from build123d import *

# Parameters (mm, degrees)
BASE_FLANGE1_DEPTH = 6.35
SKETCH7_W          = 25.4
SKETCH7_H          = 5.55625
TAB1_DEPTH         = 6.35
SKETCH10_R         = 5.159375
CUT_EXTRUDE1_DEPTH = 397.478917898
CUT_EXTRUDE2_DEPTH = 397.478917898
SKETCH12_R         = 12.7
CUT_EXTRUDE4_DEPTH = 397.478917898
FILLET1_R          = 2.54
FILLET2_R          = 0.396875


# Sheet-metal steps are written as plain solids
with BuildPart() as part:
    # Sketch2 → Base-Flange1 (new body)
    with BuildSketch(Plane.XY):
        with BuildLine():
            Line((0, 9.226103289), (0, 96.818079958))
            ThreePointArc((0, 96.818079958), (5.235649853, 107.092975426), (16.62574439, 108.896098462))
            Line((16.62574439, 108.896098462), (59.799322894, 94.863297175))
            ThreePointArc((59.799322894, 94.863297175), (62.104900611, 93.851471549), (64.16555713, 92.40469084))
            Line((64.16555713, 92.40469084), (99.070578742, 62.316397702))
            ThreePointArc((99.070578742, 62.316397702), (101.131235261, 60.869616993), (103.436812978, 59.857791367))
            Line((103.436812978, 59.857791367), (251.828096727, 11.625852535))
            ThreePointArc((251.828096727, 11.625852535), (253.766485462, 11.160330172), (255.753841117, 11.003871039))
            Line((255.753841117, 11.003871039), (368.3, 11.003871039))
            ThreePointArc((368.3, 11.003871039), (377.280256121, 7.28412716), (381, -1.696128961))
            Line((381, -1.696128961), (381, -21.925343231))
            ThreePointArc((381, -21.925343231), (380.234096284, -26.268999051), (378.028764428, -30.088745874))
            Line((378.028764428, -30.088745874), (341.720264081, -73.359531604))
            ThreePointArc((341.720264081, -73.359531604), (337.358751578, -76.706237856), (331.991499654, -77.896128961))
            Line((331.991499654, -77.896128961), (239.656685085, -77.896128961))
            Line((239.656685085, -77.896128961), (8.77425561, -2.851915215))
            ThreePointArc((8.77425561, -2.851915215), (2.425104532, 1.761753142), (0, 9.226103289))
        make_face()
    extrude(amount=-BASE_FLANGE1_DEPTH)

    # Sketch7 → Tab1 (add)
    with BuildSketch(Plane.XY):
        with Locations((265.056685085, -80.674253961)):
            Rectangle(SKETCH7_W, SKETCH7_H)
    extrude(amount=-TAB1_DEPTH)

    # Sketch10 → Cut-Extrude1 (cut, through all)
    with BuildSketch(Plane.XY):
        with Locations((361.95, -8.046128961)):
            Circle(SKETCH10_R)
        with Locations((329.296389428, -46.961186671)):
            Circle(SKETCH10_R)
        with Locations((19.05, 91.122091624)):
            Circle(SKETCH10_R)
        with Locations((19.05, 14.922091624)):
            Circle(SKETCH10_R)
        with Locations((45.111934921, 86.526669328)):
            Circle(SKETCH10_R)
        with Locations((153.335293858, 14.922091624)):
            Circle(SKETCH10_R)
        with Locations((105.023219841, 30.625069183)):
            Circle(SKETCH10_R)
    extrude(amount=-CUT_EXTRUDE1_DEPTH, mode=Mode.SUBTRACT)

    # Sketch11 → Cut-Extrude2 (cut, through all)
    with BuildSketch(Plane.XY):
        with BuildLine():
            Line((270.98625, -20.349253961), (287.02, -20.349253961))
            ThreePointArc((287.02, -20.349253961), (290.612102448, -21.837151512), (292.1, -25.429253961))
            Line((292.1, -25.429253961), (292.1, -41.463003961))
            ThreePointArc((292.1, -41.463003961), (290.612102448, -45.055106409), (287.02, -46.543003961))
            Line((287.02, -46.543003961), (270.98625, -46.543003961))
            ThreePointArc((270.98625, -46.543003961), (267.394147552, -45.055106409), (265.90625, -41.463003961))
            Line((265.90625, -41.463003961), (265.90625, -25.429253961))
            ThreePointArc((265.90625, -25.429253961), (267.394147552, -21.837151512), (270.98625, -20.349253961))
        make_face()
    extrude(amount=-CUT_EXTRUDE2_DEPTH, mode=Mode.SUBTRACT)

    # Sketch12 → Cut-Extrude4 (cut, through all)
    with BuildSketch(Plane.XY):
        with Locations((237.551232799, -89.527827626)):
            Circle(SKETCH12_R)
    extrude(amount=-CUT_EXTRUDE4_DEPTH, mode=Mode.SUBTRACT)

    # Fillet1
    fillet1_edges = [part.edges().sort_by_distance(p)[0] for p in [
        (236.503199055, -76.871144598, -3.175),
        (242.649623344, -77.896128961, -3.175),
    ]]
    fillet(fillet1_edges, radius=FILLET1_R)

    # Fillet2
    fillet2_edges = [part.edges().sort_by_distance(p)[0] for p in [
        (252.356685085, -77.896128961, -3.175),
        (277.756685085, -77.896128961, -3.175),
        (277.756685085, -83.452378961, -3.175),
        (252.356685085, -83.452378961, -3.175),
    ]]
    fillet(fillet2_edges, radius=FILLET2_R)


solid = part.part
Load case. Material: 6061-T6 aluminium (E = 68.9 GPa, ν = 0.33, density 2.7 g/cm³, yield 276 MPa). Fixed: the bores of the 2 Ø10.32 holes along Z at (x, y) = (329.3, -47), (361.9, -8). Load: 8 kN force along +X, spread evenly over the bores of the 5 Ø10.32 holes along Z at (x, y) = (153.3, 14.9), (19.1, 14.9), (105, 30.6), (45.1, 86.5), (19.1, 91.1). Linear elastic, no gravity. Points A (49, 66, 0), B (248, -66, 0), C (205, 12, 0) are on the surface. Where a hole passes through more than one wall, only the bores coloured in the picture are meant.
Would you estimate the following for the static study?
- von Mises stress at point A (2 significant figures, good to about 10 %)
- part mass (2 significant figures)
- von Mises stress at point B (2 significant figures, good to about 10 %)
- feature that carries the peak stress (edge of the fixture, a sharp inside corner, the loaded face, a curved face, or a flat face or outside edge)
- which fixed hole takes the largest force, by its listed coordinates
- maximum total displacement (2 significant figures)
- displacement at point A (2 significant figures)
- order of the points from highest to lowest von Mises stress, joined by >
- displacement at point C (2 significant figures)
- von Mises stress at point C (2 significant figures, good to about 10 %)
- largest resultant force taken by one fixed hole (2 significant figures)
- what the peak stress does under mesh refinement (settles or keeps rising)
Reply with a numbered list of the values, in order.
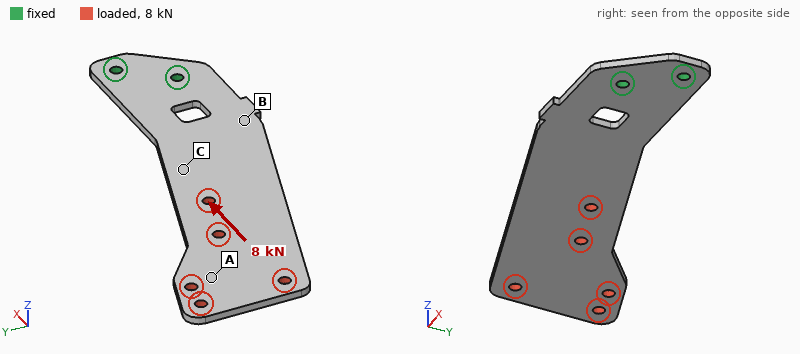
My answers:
1. 14 MPa
2. 590 g
3. 36 MPa
4. edge of the fixture
5. (361.9, -8)
6. 1.7 mm
7. 1.3 mm
8. C > B > A
9. 0.40 mm
10. 56 MPa
11. 14 kN
12. keeps rising
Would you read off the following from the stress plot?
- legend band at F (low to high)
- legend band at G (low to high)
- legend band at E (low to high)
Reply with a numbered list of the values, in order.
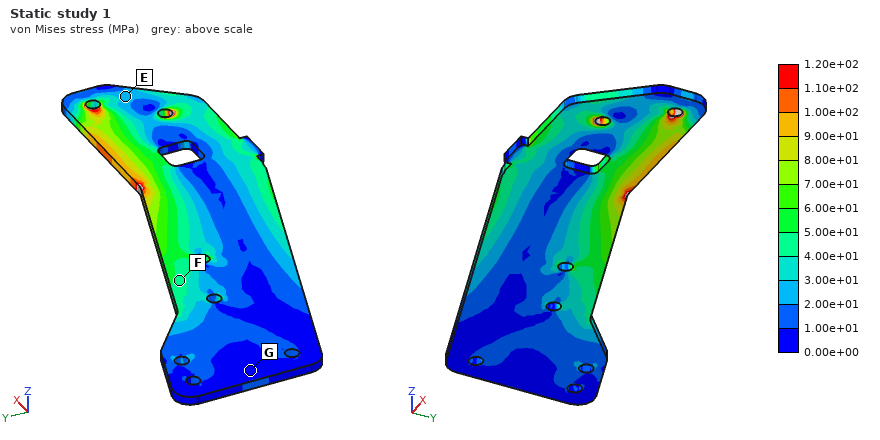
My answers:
1. 4.00e+01 to 5.00e+01 MPa
2. 0.00e+00 to 1.00e+01 MPa
3. 2.00e+01 to 3.00e+01 MPa
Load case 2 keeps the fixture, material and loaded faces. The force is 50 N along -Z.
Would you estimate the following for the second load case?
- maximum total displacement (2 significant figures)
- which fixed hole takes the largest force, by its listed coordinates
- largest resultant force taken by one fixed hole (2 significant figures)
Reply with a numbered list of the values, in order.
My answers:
1. 4.4 mm
2. (329.3, -47)
3. 120 N
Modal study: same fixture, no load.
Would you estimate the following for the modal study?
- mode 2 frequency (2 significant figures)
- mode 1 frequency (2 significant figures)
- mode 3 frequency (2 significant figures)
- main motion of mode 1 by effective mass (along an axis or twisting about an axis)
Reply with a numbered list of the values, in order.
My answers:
1. 230 Hz
2. 39 Hz
3. 310 Hz
4. along Z
